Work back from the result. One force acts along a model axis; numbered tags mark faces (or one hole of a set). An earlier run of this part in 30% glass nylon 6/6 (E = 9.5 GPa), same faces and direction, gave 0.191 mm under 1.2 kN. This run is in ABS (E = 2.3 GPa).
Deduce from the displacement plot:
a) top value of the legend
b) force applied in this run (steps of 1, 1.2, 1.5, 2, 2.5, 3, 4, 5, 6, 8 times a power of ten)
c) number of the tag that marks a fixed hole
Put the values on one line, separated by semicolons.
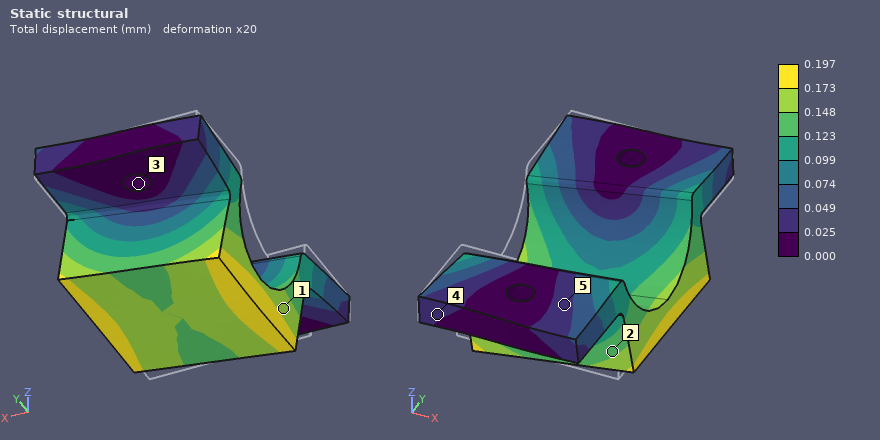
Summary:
0.197 mm; 300 N; 3
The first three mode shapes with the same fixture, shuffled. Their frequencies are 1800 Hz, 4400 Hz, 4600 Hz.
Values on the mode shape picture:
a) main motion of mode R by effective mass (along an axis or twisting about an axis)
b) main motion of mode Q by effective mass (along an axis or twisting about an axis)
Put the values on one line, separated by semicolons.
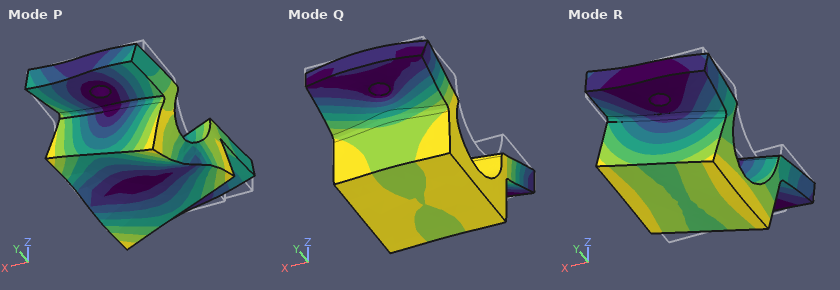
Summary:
along X; along Z
